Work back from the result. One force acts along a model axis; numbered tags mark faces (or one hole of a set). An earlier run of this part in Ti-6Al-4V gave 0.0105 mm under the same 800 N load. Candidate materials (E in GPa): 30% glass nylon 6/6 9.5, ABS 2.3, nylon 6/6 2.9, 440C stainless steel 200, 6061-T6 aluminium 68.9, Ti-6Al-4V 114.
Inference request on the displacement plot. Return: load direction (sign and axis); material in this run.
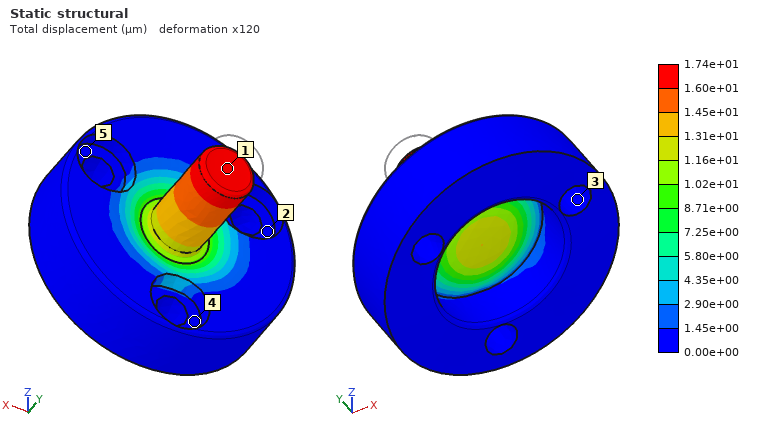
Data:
-Y
6061-T6 aluminium
